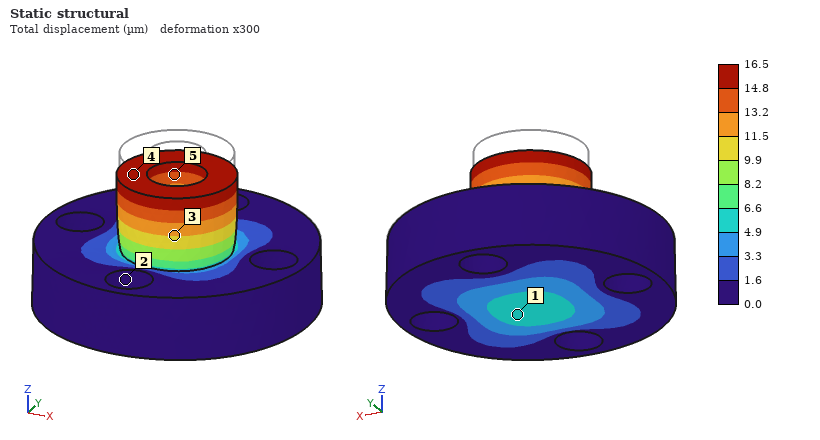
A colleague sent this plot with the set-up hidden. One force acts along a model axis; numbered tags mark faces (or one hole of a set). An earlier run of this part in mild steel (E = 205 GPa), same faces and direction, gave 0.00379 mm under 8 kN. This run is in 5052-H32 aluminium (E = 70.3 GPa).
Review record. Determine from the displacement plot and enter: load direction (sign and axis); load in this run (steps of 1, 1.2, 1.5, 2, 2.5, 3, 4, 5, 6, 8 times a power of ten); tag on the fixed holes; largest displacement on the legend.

-Z
12 kN
2
16.5 µm
